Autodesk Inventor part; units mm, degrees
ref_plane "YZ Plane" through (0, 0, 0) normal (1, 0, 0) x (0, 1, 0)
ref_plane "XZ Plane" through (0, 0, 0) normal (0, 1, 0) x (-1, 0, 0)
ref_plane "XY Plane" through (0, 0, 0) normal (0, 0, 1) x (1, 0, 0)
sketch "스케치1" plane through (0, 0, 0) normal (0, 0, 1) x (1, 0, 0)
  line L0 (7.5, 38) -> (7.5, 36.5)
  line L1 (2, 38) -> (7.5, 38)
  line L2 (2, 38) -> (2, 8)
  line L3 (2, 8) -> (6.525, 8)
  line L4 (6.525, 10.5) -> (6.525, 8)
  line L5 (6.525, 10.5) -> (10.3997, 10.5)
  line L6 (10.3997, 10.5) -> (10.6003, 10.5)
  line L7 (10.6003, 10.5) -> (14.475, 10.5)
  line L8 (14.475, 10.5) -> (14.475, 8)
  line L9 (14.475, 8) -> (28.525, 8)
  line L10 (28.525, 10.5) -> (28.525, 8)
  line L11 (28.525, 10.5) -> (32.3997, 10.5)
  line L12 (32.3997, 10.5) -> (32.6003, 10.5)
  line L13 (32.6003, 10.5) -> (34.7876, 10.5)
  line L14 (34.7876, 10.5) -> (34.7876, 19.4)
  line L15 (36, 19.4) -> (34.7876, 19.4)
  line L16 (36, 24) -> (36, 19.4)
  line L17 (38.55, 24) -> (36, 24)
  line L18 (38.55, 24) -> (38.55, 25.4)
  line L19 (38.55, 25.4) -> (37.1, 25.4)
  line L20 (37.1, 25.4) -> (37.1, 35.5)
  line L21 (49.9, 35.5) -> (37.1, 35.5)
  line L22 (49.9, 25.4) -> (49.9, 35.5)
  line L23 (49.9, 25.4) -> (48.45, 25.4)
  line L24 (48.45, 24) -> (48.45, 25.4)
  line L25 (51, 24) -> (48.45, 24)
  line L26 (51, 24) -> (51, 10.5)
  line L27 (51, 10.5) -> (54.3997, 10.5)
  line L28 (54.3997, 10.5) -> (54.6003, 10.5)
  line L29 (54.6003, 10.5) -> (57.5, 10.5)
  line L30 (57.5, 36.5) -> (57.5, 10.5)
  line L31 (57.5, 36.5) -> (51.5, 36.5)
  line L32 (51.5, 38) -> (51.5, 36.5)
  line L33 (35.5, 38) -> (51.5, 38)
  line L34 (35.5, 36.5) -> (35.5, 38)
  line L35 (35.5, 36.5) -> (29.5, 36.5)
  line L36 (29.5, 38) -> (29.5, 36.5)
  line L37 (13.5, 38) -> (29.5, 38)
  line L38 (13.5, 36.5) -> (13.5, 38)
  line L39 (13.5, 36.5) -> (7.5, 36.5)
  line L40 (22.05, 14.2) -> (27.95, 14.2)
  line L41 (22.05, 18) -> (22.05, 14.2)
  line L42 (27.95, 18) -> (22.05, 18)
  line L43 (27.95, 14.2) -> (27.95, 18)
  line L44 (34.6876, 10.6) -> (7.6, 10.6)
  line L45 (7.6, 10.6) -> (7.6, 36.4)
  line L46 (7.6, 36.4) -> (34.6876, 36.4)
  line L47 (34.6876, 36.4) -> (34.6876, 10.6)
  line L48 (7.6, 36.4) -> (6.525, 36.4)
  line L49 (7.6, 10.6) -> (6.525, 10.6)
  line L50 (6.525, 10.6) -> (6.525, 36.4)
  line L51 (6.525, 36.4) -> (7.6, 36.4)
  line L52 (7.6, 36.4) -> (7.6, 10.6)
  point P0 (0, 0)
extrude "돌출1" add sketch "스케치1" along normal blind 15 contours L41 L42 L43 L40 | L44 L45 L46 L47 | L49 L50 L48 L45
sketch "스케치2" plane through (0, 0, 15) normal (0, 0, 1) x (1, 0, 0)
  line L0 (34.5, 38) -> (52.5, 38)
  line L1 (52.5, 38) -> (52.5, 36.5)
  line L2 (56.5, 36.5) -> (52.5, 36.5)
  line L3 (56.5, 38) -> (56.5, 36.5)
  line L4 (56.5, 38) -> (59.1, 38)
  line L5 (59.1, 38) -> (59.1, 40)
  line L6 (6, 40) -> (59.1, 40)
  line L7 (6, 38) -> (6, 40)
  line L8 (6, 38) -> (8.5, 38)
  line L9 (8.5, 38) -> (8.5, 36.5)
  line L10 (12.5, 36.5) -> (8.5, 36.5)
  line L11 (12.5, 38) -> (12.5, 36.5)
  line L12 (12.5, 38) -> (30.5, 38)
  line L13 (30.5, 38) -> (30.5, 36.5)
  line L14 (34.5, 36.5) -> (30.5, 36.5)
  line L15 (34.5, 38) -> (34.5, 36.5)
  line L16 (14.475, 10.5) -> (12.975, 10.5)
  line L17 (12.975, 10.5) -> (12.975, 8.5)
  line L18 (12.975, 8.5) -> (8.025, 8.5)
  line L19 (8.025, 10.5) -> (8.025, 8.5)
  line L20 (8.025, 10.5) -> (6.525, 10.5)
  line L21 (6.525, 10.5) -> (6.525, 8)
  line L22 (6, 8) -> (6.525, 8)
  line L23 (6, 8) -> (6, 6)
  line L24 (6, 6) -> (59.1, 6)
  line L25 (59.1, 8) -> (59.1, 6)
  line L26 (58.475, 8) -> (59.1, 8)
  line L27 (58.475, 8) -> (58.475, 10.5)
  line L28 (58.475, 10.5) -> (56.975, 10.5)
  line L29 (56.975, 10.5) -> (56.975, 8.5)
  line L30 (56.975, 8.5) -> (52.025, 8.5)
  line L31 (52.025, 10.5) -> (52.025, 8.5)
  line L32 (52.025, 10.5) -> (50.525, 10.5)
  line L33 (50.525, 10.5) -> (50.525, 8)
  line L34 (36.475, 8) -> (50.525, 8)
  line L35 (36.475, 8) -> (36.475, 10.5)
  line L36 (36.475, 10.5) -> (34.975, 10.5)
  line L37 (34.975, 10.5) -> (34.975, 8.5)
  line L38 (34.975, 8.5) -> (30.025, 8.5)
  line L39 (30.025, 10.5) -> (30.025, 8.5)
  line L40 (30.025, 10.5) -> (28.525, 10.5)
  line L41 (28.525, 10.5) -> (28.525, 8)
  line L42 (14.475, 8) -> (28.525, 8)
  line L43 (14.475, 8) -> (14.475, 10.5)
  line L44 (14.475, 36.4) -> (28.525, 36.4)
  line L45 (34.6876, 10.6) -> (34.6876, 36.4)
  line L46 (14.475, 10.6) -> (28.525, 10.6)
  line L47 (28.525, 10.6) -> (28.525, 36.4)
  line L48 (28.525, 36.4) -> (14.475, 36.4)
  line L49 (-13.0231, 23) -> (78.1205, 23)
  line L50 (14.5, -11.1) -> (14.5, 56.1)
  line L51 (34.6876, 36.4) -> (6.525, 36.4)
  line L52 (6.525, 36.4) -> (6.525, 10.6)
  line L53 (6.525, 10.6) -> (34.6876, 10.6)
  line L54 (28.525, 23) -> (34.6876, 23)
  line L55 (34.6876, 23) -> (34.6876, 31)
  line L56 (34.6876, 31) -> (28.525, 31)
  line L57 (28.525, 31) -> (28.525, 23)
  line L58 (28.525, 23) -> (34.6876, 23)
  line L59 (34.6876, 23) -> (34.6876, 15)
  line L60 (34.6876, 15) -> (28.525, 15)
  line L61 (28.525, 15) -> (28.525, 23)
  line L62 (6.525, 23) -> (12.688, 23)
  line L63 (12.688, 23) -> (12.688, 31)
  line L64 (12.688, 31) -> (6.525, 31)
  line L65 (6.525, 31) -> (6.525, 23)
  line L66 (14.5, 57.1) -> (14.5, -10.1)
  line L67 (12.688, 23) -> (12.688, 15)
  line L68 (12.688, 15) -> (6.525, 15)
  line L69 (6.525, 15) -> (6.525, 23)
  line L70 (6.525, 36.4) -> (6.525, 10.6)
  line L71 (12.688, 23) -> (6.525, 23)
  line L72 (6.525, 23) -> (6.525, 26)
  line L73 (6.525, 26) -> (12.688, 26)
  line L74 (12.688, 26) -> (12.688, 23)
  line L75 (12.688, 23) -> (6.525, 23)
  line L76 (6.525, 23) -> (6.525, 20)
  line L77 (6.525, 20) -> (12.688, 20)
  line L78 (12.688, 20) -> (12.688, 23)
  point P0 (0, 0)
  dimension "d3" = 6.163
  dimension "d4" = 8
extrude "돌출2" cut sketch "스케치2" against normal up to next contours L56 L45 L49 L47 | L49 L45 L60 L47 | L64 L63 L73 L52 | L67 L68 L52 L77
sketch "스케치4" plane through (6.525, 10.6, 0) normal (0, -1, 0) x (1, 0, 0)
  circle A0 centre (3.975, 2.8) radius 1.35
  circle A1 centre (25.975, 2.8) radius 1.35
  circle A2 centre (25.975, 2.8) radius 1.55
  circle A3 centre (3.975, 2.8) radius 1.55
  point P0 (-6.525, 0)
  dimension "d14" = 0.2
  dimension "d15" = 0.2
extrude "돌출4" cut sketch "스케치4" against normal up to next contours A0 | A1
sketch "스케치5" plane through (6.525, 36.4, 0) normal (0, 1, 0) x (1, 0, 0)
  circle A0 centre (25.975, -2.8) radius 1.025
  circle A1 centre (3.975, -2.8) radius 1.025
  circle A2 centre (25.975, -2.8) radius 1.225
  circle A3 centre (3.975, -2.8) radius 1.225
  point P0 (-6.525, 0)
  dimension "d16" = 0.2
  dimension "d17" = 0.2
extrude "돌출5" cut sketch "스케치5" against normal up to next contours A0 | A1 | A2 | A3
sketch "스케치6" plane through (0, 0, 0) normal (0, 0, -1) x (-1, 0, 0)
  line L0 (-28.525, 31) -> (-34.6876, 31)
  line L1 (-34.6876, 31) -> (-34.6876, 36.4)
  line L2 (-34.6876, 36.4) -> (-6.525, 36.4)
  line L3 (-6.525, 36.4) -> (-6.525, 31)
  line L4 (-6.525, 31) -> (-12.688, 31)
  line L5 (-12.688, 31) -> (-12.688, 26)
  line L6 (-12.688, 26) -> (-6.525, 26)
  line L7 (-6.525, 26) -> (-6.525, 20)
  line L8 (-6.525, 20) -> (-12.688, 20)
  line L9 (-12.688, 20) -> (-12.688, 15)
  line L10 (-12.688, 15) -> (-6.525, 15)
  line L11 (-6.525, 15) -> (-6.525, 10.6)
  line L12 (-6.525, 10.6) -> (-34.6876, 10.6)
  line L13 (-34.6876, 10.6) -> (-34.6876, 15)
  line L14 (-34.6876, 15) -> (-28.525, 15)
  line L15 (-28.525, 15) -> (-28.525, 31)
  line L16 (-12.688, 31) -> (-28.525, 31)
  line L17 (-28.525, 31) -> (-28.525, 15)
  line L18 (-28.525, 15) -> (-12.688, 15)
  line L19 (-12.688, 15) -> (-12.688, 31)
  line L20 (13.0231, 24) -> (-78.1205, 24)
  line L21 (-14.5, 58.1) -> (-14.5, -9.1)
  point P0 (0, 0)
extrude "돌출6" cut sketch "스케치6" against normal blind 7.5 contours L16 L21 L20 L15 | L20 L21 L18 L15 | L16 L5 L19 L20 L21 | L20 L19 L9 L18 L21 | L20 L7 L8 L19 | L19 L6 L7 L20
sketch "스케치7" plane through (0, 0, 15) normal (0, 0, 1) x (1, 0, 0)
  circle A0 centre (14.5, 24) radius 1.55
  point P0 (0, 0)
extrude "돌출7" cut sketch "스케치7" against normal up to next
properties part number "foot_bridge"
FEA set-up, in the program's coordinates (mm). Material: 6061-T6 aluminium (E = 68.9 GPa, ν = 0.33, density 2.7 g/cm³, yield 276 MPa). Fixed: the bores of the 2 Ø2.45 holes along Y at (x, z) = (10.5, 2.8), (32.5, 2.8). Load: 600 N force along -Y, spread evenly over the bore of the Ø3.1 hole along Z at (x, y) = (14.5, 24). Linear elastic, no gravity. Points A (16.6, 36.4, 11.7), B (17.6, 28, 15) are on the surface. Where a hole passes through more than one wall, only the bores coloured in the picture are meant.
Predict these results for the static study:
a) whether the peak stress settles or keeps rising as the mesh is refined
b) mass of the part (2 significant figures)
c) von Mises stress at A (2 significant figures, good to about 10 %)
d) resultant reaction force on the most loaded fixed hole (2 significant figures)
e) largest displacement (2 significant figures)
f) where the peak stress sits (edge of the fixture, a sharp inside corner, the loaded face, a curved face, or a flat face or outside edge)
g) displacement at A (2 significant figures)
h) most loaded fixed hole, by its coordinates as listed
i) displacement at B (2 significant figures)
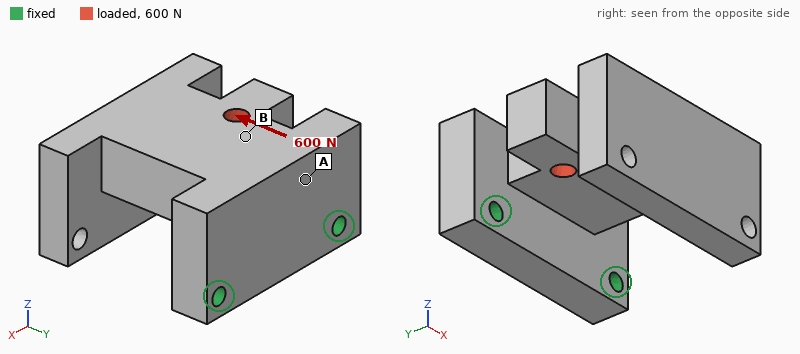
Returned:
keeps rising
17 g
17 MPa
500 N
45 µm
edge of the fixture
15 µm
(10.5, 2.8)
21 µm
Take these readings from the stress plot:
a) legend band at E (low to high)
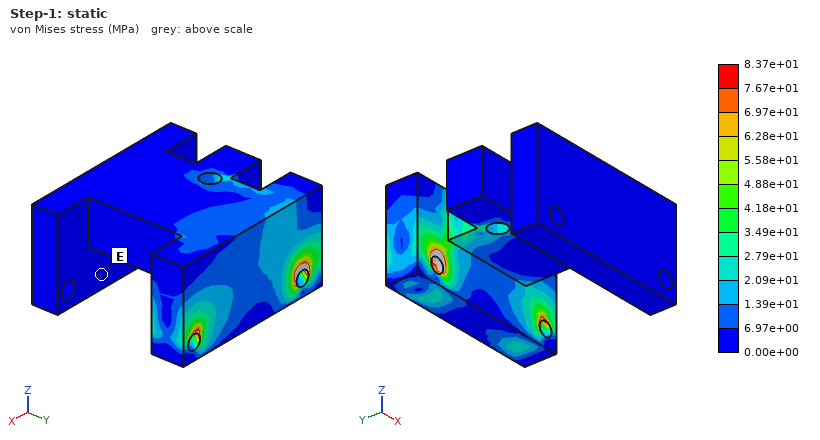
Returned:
0.00e+00 to 6.97e+00 MPa
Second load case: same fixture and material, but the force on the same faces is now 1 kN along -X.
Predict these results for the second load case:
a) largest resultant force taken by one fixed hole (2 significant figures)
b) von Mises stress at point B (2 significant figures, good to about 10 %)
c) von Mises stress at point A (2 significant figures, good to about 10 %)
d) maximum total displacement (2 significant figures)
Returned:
780 N
12 MPa
14 MPa
34 µm
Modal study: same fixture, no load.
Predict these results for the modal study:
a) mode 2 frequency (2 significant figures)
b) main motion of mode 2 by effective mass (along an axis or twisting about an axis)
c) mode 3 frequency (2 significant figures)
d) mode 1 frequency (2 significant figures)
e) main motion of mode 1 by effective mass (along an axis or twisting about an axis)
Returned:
6800 Hz
along X
11 kHz
3700 Hz
along Z
